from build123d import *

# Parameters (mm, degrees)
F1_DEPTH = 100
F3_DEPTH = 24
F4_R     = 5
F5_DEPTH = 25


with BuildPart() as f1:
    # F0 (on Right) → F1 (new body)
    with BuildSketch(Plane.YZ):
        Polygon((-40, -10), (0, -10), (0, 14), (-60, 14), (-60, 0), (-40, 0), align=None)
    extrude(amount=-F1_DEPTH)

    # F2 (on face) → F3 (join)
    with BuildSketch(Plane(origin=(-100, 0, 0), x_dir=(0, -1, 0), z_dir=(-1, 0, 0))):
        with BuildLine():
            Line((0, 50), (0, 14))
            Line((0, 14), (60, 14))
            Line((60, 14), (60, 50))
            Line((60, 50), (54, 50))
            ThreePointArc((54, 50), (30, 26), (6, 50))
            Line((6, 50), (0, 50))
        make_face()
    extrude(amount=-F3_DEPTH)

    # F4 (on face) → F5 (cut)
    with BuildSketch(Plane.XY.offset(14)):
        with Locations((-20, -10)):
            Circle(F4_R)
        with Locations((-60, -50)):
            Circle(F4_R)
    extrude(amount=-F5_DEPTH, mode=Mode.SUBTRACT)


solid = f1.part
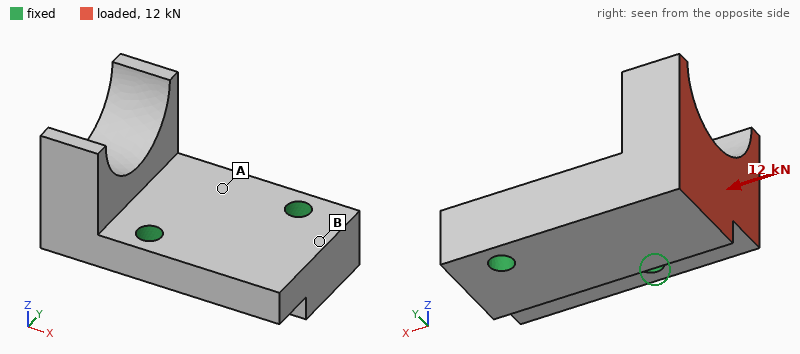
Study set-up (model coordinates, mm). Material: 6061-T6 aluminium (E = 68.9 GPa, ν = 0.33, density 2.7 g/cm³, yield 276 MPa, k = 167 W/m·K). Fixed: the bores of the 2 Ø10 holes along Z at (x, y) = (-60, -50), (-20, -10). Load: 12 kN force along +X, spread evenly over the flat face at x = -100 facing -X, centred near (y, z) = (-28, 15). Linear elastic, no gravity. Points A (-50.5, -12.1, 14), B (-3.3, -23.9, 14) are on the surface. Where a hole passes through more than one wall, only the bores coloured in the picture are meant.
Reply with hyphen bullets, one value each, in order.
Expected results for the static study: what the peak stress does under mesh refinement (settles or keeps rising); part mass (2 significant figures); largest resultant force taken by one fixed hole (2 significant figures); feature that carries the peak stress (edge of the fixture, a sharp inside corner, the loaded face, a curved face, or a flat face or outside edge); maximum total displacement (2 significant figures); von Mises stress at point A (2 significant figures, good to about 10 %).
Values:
- keeps rising
- 410 g
- 6.4 kN
- edge of the fixture
- 0.12 mm
- 28 MPa
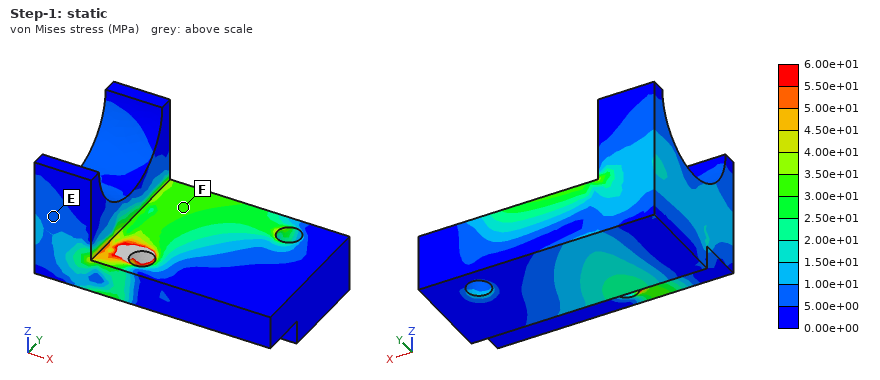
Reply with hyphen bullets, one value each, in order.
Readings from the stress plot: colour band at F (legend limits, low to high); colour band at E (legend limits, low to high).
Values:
- 3.00e+01 to 3.50e+01 MPa
- 5.00e+00 to 1.00e+01 MPa
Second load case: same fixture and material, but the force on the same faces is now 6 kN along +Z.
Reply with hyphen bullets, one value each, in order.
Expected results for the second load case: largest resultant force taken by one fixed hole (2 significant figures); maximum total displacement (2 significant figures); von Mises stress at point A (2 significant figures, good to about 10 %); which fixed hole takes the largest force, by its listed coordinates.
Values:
- 6.3 kN
- 0.20 mm
- 37 MPa
- (-60, -50)
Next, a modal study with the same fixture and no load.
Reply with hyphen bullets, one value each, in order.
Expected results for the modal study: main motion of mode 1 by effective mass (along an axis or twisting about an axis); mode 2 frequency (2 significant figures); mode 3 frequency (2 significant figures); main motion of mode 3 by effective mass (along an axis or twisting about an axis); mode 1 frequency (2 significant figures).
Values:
- along Z
- 5500 Hz
- 8100 Hz
- along Y
- 3100 Hz
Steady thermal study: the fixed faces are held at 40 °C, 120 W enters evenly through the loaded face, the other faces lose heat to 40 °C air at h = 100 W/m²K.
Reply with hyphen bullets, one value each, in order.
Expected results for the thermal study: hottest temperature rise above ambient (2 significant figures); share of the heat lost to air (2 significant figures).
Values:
- 26 K
- 18 %
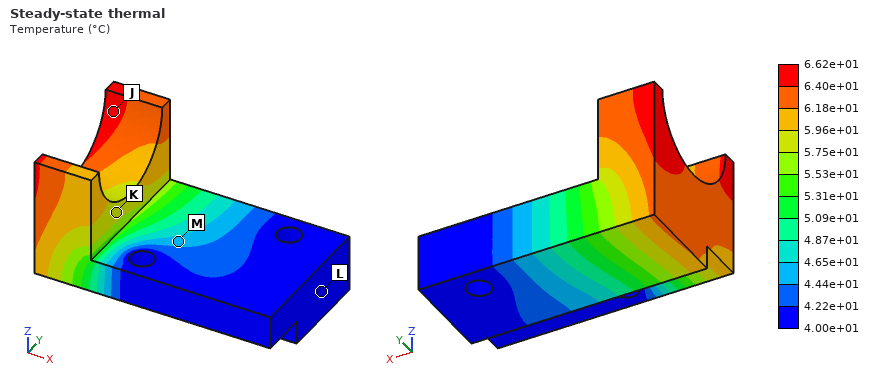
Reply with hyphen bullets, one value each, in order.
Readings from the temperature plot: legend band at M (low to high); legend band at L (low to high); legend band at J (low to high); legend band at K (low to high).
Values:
- 4.44e+01 to 4.65e+01 °C
- 4.00e+01 to 4.22e+01 °C
- 6.40e+01 to 6.62e+01 °C
- 5.75e+01 to 5.96e+01 °C
